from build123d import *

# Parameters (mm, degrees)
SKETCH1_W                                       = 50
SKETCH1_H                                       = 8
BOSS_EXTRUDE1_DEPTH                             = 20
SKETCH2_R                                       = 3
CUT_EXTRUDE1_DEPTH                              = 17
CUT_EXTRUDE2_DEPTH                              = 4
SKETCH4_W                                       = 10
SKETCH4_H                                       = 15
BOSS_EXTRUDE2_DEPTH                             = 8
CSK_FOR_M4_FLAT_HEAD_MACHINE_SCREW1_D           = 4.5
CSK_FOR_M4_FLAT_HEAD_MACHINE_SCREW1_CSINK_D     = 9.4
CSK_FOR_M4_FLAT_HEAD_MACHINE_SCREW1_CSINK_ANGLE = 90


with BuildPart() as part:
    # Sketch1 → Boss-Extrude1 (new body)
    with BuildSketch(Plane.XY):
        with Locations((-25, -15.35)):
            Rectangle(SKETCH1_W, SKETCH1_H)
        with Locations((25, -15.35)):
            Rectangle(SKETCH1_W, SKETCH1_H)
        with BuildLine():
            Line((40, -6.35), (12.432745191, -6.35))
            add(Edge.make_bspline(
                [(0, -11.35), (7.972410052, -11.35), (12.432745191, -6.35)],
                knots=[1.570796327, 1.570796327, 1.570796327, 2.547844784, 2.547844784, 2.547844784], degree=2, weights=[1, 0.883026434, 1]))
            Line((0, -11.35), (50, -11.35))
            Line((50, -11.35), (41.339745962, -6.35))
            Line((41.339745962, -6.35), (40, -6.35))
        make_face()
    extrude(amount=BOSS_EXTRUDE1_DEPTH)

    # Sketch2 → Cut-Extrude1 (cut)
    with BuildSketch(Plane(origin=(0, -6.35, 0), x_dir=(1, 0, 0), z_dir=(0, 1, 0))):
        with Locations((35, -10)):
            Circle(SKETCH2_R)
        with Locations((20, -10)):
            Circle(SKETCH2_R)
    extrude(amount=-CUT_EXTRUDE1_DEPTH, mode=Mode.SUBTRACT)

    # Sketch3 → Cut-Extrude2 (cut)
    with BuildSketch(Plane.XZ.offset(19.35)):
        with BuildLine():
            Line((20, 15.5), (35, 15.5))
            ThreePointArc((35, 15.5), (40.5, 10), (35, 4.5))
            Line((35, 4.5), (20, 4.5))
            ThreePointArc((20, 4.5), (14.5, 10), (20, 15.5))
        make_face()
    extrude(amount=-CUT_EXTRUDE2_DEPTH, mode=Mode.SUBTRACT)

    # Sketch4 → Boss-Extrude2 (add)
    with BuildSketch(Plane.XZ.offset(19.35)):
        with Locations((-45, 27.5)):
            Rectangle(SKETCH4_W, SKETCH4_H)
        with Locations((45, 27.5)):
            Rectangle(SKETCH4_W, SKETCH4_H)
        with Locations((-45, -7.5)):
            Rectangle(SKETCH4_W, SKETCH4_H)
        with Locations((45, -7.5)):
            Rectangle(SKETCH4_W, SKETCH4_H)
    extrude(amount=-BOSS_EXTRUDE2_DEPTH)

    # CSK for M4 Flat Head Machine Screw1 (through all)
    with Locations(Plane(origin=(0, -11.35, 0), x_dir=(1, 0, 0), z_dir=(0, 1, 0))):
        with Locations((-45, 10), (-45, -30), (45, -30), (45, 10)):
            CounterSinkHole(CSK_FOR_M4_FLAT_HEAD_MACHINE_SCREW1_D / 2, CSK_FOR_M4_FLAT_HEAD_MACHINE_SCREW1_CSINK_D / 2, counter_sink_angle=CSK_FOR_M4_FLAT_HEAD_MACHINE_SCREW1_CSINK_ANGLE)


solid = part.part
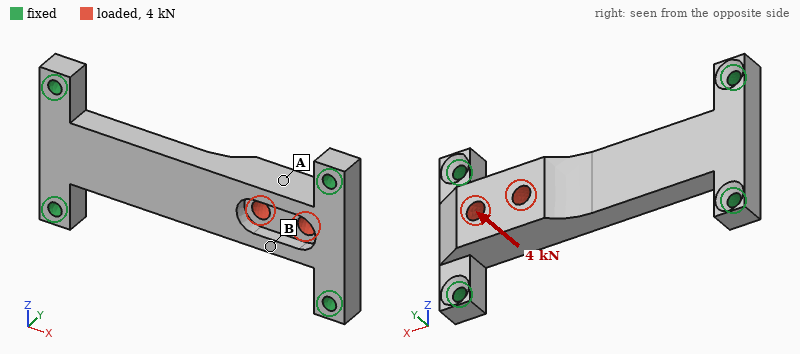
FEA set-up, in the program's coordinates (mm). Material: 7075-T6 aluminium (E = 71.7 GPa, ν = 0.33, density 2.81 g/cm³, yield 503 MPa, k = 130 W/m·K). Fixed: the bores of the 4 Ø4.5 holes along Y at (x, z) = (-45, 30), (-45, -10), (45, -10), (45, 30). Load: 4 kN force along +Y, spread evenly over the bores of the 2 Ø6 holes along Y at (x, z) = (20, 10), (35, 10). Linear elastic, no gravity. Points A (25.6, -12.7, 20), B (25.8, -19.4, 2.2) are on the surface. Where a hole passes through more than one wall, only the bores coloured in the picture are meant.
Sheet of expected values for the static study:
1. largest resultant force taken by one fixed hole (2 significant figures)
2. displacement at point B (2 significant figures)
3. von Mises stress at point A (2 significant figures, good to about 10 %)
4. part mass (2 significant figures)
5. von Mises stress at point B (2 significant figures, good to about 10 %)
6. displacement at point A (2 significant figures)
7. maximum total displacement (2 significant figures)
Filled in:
2.0 kN
0.13 mm
28 MPa
62 g
69 MPa
0.13 mm
0.19 mm
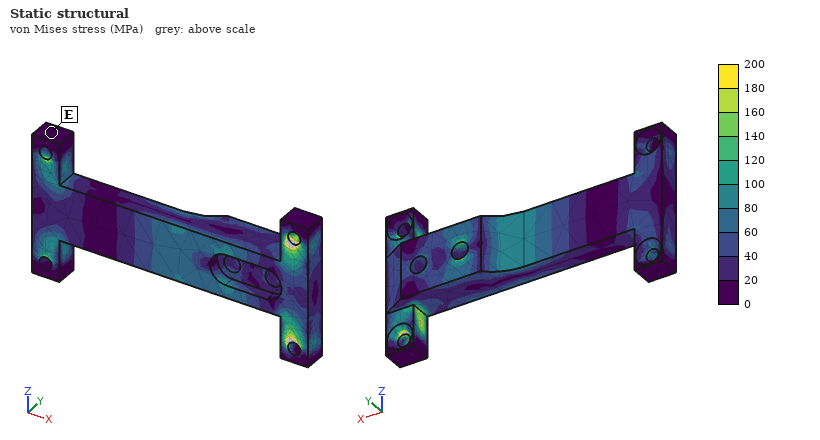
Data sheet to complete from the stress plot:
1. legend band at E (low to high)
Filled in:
0 to 20 MPa
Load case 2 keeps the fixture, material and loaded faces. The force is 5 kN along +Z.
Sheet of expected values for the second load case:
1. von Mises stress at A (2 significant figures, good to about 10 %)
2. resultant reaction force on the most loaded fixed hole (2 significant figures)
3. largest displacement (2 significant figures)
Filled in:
30 MPa
2.6 kN
49 µm
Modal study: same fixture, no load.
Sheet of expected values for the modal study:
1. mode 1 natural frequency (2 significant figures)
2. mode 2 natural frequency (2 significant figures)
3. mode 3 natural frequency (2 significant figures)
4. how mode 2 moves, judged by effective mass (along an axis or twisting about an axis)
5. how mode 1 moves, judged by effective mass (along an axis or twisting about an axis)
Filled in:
3400 Hz
8100 Hz
10 kHz
along Z
along Y
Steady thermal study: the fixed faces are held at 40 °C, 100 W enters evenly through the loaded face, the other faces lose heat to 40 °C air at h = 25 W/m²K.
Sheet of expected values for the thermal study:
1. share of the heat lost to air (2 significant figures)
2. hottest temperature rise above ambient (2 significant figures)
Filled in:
7.9 %
81 K
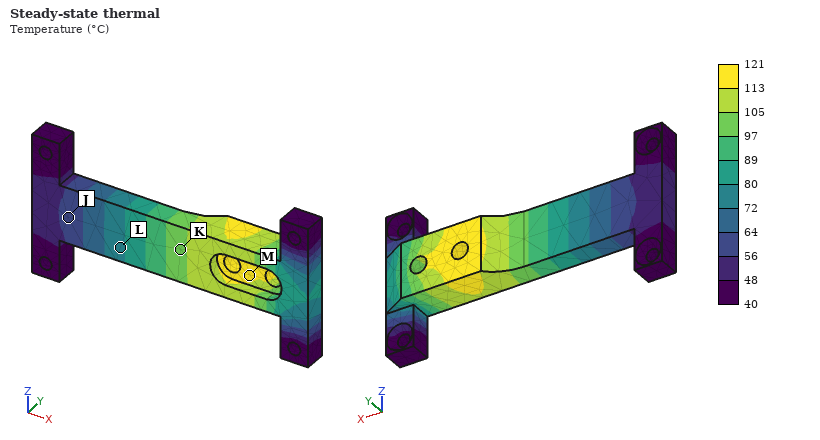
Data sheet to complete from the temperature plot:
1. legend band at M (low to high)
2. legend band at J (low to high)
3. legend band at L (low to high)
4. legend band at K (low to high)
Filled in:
113 to 121 °C
56 to 64 °C
72 to 80 °C
97 to 105 °C
